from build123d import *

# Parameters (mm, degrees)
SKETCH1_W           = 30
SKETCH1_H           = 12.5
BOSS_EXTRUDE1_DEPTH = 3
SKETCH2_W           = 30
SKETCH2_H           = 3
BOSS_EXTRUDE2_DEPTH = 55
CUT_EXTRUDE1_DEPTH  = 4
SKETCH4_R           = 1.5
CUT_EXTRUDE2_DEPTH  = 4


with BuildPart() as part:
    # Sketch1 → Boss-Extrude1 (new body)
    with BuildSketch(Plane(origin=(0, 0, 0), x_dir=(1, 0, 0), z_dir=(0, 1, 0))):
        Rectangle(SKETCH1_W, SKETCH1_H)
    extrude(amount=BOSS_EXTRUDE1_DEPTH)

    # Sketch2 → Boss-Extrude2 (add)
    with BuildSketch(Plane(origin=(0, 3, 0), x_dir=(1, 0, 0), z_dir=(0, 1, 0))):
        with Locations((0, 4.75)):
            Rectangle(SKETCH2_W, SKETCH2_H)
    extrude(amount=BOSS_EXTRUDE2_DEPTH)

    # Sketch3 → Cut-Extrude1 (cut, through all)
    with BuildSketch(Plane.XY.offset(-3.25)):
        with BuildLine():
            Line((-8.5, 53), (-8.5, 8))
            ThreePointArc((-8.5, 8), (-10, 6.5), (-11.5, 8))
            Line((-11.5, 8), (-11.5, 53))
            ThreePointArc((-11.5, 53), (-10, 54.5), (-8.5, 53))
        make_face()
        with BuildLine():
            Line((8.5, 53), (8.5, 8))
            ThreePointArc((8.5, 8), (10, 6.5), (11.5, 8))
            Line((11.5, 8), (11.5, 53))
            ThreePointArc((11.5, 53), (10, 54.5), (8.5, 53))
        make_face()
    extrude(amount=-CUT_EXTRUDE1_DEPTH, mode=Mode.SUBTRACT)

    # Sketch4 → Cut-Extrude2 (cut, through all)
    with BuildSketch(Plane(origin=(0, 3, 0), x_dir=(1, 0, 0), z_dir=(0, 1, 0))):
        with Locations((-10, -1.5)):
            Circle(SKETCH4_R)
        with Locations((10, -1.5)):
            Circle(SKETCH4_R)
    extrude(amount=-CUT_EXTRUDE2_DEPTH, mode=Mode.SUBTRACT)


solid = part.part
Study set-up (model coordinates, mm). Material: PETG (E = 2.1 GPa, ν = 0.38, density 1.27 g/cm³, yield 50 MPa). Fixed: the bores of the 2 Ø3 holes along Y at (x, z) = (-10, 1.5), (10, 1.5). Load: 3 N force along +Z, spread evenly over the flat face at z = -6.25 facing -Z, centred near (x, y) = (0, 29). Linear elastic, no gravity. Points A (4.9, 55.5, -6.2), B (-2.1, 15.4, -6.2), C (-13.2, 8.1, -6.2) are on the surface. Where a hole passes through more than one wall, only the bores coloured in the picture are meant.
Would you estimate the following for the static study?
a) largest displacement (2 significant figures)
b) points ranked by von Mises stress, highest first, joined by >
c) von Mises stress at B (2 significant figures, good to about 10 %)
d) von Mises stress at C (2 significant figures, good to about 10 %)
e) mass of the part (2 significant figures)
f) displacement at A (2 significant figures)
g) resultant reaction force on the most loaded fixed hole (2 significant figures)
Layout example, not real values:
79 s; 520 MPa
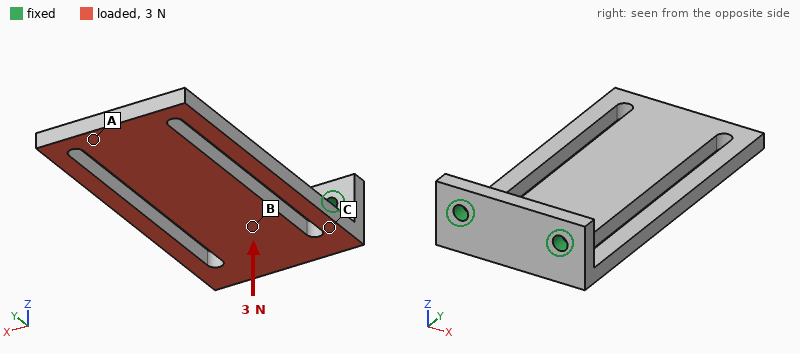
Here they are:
0.70 mm; C > B > A; 1.2 MPa; 1.8 MPa; 6.6 g; 0.66 mm; 1.6 N
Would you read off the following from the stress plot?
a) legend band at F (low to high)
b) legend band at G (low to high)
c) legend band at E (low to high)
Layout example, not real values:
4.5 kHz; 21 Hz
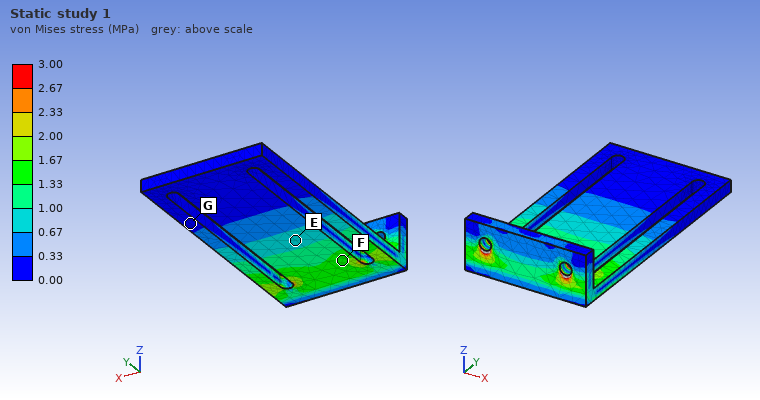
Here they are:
1.33 to 1.67 MPa; 0.00 to 0.33 MPa; 0.67 to 1.00 MPa
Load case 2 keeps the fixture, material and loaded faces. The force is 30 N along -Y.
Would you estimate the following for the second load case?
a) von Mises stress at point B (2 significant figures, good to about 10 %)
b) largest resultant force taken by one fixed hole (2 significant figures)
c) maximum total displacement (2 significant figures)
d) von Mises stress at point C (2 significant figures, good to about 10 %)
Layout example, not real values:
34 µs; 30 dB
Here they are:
1.1 MPa; 15 N; 0.72 mm; 1.4 MPa
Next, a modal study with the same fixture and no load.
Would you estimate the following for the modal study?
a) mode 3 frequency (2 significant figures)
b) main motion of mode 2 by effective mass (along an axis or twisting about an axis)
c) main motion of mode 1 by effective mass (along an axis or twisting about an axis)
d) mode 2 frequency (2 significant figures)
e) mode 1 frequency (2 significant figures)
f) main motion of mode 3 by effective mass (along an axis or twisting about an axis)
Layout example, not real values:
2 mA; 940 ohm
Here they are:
770 Hz; along X; along Z; 630 Hz; 170 Hz; along X
